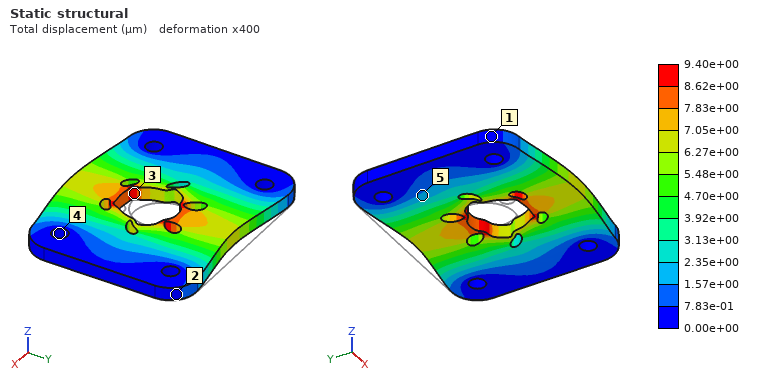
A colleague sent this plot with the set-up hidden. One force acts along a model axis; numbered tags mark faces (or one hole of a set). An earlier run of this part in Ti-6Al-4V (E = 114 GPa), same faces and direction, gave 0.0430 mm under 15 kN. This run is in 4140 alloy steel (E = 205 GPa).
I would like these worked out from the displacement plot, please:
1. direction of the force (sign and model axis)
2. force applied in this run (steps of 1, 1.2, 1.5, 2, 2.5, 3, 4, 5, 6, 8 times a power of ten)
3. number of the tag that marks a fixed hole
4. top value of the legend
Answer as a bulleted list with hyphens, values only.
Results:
- -Y
- 6 kN
- 4
- 9.40e+00 µm
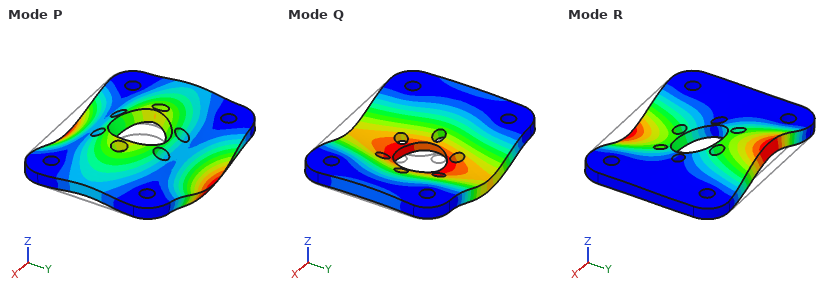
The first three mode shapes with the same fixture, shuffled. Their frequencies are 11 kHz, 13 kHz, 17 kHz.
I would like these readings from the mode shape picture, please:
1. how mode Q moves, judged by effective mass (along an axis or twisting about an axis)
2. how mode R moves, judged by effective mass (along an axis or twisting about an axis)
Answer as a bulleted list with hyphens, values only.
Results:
- along Z
- twisting about X
